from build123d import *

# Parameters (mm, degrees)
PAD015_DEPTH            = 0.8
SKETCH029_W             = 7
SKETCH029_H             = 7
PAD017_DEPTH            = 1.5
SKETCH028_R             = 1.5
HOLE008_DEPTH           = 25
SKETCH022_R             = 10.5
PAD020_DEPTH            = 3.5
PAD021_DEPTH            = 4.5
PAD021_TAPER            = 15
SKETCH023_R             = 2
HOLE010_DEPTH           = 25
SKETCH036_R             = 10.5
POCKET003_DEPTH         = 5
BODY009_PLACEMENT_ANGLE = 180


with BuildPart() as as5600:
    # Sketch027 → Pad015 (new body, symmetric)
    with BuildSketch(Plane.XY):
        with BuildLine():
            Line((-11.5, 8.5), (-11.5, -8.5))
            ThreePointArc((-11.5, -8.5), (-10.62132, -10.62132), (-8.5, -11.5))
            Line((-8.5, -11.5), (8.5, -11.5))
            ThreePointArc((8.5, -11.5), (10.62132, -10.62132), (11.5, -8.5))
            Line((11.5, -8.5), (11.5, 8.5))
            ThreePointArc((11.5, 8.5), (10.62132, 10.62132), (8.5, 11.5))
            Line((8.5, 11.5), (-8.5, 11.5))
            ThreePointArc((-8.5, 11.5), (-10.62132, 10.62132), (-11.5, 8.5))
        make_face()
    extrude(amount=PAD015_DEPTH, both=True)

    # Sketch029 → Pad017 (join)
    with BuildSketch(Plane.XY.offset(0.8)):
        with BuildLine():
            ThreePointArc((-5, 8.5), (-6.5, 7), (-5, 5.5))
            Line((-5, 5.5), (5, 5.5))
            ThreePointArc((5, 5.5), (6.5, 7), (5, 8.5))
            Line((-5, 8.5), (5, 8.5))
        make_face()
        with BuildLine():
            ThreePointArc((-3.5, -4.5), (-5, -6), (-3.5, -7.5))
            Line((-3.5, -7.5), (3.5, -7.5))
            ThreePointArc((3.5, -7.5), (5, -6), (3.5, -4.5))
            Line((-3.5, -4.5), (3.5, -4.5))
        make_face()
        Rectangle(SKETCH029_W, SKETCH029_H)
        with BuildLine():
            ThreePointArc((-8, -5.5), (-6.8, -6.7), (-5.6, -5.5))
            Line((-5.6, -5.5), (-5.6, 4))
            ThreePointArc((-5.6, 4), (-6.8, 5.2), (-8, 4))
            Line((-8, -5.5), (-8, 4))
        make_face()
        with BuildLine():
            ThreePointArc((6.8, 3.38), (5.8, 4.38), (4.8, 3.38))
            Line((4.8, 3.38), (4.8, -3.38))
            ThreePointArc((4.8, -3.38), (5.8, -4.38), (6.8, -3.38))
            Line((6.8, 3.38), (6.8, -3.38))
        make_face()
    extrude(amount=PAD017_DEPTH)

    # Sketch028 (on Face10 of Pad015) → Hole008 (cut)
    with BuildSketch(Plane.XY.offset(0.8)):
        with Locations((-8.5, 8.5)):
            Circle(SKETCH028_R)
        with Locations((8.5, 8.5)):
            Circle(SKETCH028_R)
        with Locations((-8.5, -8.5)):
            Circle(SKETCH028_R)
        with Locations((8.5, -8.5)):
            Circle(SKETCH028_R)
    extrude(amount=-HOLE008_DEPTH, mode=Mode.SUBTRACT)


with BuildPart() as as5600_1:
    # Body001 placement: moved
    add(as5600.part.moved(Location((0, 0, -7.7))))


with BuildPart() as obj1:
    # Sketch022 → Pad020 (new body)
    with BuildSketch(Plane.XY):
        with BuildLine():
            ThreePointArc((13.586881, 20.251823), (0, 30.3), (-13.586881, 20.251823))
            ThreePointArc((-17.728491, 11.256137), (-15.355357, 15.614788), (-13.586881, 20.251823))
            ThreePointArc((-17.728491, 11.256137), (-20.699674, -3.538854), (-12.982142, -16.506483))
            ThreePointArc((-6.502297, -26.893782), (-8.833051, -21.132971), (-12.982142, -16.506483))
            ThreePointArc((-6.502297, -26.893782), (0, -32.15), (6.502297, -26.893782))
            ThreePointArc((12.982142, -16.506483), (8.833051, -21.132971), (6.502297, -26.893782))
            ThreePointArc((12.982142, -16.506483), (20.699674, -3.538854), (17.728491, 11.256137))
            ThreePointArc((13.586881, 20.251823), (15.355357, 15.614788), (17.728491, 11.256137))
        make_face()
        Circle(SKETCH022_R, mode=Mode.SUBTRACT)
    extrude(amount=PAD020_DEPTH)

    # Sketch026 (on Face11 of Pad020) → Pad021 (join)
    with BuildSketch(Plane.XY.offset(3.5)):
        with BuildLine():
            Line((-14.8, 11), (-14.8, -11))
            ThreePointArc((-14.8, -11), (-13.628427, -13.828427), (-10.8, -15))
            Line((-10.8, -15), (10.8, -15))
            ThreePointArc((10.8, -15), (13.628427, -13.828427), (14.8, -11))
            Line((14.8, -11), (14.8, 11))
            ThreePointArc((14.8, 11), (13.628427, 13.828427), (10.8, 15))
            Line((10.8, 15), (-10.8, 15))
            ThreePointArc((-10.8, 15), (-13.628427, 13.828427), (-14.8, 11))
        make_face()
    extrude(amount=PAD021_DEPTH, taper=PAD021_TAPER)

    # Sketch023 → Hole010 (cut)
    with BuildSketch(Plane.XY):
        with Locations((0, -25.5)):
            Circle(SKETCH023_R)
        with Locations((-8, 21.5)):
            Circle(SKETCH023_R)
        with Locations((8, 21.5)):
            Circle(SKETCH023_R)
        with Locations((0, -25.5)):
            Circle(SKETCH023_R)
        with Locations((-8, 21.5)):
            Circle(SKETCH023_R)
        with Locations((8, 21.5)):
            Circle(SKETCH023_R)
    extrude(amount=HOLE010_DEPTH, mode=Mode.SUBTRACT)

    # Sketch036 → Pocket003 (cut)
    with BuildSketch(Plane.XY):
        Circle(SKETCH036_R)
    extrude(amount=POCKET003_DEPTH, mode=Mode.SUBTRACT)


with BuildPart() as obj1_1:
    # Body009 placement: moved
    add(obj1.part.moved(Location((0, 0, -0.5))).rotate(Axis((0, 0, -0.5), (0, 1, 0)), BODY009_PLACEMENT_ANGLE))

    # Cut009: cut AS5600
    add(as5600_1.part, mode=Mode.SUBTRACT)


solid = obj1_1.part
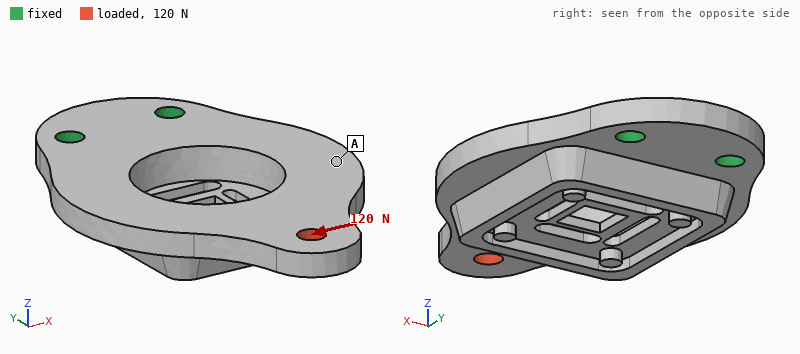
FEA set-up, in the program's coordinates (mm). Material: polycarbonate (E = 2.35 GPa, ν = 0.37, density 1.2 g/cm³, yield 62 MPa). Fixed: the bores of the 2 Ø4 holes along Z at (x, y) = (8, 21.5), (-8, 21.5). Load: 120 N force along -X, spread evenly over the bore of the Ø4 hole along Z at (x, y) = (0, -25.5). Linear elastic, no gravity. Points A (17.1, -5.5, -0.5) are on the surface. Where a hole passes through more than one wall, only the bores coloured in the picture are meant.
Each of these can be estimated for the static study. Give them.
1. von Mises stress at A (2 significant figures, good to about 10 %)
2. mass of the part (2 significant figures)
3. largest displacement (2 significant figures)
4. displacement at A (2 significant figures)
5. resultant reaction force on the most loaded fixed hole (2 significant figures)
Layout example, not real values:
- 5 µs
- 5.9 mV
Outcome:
- 2.5 MPa
- 8.4 g
- 0.54 mm
- 0.36 mm
- 300 N
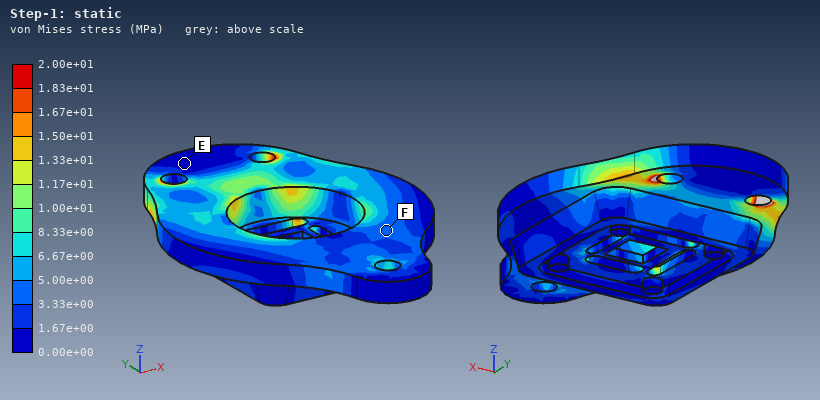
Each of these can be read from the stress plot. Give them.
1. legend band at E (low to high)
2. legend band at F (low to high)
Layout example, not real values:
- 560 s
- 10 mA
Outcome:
- 0.00e+00 to 1.67e+00 MPa
- 3.33e+00 to 5.00e+00 MPa
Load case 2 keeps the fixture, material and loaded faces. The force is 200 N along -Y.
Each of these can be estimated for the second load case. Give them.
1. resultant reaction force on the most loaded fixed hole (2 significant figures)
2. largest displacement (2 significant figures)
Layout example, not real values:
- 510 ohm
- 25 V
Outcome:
- 100 N
- 0.40 mm
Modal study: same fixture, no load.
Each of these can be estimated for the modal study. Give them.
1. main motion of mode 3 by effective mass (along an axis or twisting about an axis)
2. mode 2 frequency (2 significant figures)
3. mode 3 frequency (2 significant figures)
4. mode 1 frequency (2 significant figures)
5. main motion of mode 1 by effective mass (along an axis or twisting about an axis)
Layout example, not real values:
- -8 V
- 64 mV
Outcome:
- along X
- 1300 Hz
- 1700 Hz
- 420 Hz
- along Z
